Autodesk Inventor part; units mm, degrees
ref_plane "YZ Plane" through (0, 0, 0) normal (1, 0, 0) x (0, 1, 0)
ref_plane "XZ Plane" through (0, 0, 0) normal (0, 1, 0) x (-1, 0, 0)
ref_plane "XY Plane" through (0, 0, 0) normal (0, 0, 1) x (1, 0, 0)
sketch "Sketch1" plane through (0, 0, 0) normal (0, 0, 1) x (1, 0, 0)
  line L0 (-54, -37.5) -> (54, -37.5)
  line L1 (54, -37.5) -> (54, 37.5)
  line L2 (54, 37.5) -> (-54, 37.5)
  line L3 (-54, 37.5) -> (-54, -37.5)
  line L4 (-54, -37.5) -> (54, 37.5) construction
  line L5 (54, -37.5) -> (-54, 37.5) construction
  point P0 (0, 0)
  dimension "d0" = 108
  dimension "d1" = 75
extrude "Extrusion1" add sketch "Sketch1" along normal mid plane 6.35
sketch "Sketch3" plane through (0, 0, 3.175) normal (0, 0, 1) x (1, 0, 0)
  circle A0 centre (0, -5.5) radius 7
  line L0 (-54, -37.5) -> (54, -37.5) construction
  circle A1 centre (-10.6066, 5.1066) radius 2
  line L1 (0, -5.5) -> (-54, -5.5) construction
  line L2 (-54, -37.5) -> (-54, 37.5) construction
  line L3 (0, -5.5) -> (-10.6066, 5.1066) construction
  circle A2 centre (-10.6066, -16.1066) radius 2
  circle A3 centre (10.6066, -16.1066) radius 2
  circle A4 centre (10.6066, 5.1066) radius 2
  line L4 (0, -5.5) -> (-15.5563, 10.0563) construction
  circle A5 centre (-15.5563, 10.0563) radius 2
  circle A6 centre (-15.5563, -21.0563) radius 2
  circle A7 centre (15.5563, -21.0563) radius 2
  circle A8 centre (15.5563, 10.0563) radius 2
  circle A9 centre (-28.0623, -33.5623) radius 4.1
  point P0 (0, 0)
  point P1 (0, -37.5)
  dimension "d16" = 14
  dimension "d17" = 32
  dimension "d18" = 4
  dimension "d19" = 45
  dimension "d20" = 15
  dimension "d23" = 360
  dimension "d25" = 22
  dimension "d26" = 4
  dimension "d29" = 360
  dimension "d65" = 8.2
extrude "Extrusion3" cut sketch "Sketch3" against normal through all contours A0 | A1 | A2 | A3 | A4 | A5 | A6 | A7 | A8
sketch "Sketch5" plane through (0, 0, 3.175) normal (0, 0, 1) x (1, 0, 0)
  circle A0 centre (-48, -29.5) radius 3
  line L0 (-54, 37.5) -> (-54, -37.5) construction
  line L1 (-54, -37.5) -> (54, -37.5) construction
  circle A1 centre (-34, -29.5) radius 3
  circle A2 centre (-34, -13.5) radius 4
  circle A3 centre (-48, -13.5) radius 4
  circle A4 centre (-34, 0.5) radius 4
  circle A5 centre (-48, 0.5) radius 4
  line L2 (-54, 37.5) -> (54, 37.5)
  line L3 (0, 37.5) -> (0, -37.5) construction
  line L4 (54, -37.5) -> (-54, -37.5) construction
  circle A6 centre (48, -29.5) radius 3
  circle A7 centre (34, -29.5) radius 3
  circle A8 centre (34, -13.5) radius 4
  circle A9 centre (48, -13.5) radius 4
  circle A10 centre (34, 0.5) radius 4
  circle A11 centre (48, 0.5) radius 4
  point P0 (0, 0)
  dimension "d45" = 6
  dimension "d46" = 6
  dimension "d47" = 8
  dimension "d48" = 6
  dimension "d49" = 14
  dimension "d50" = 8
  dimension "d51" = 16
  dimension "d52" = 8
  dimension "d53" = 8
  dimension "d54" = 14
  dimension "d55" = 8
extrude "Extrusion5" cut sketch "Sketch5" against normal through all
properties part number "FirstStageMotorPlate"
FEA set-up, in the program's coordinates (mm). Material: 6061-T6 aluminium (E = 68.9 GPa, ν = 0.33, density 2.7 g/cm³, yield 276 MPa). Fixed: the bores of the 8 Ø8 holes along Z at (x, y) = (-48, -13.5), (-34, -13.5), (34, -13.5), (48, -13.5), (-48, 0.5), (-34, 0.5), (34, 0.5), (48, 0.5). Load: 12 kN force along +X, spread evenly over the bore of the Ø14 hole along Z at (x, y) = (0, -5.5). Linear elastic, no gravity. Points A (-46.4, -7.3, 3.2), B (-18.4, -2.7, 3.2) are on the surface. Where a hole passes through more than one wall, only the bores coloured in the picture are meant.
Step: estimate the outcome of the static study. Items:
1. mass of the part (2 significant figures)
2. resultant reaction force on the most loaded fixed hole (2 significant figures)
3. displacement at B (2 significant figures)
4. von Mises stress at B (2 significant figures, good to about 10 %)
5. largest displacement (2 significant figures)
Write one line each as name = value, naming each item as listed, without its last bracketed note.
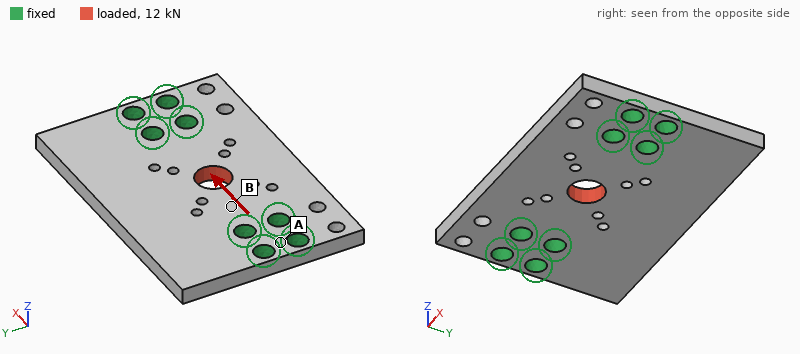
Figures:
mass of the part = 130 g
resultant reaction force on the most loaded fixed hole = 2.9 kN
displacement at B = 6.1 µm
von Mises stress at B = 38 MPa
largest displacement = 15 µm
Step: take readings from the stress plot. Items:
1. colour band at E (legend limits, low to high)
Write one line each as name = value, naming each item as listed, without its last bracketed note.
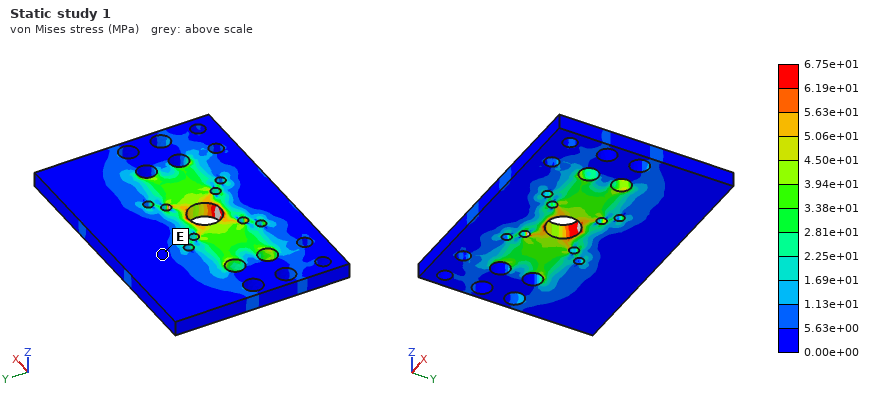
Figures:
colour band at E = 0.00e+00 to 5.63e+00 MPa
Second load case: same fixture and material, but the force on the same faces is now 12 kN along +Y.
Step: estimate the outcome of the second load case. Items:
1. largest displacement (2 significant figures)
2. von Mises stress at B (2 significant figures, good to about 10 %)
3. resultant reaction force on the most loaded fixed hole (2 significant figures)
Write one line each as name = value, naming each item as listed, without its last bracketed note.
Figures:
largest displacement = 27 µm
von Mises stress at B = 31 MPa
resultant reaction force on the most loaded fixed hole = 3.5 kN
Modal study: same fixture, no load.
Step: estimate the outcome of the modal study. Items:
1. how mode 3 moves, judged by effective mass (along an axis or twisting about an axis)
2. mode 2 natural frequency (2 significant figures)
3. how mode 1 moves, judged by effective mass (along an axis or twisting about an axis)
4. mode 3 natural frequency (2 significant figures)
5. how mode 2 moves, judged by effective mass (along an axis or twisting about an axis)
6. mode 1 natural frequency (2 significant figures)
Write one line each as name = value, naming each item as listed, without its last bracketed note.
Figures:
how mode 3 moves, judged by effective mass = along Z
mode 2 natural frequency = 5300 Hz
how mode 1 moves, judged by effective mass = along Z
mode 3 natural frequency = 6000 Hz
how mode 2 moves, judged by effective mass = twisting about Y
mode 1 natural frequency = 3400 Hz
